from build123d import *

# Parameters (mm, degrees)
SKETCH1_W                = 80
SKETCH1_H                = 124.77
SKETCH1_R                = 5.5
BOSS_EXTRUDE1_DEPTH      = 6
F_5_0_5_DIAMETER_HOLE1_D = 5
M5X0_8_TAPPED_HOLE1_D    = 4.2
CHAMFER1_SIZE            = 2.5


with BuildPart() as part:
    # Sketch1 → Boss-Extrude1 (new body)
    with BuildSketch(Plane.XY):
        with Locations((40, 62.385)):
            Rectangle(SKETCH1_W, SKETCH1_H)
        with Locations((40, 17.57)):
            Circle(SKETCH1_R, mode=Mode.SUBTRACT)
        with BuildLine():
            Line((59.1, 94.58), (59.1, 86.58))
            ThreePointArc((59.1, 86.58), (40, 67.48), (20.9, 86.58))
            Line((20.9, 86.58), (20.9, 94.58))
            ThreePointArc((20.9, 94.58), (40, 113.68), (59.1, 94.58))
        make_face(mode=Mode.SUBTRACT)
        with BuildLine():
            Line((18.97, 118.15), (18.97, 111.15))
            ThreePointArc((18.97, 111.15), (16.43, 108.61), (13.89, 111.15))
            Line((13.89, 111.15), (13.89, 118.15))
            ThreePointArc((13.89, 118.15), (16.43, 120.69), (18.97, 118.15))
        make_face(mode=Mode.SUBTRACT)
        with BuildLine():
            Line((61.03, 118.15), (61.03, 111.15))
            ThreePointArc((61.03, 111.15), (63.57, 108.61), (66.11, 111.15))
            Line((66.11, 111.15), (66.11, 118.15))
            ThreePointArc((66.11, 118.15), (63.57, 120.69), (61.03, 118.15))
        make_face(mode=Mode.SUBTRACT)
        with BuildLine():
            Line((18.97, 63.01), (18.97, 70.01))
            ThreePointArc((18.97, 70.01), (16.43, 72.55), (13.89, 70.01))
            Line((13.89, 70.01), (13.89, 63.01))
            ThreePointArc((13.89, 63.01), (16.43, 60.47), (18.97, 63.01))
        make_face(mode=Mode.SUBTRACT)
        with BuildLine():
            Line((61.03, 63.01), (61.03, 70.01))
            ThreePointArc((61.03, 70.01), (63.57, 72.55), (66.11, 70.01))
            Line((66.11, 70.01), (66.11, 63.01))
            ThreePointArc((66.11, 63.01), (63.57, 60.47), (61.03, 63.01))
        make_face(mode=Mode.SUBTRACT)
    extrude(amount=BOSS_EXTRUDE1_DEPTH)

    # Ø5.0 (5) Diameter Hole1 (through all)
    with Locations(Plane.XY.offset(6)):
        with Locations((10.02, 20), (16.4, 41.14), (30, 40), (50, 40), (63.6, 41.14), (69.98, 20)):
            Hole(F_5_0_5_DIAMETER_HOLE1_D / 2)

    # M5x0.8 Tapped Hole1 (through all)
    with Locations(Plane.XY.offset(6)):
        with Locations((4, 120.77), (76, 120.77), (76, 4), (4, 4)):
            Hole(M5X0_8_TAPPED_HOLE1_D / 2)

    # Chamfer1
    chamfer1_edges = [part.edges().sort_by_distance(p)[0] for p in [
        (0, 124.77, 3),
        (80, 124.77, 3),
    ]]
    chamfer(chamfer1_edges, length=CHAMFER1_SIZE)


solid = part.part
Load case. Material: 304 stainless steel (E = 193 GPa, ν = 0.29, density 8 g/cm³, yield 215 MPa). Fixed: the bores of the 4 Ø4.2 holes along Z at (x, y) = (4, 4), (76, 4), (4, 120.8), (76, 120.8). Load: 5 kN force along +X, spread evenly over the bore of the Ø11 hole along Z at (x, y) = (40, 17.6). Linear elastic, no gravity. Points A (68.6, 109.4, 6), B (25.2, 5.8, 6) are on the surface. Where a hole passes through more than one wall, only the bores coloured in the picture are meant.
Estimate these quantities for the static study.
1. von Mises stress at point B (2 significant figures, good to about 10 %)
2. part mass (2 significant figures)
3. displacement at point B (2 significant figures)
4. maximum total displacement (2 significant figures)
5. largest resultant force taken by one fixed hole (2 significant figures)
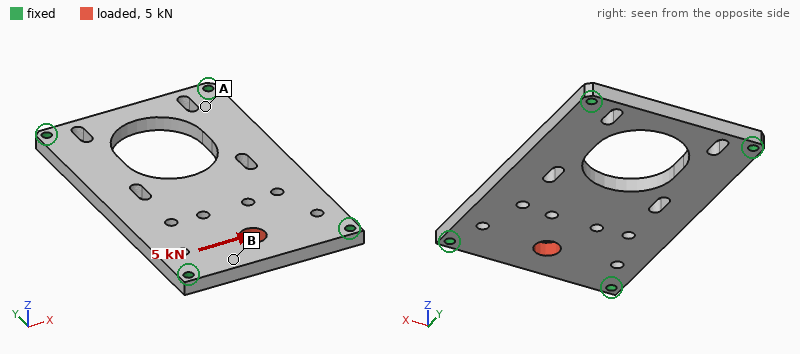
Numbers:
18 MPa
390 g
2.8 µm
5.5 µm
2.4 kN
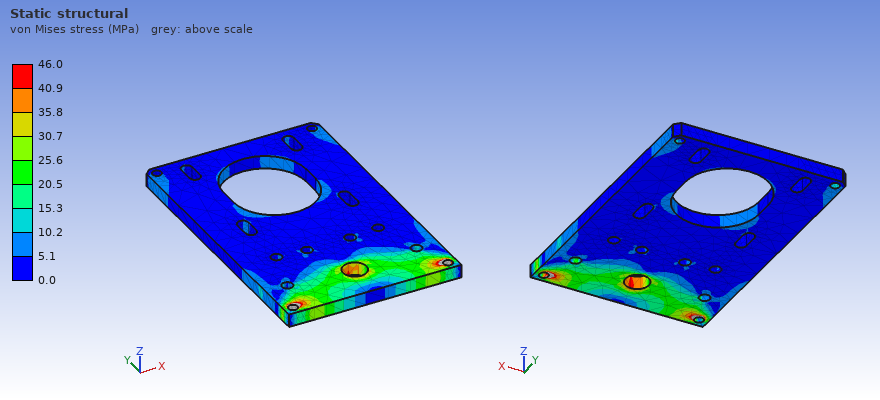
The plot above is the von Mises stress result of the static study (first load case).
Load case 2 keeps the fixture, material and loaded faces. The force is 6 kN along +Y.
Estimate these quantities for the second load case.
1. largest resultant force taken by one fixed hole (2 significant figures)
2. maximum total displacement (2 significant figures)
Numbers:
2.3 kN
9.2 µm
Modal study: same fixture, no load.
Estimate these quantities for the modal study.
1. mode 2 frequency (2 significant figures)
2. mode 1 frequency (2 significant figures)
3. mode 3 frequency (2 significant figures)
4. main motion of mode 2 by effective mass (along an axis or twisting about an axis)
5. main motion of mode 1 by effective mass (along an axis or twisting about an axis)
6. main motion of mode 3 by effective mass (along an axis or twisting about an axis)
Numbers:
2700 Hz
1700 Hz
4400 Hz
twisting about Y
along Z
twisting about X
